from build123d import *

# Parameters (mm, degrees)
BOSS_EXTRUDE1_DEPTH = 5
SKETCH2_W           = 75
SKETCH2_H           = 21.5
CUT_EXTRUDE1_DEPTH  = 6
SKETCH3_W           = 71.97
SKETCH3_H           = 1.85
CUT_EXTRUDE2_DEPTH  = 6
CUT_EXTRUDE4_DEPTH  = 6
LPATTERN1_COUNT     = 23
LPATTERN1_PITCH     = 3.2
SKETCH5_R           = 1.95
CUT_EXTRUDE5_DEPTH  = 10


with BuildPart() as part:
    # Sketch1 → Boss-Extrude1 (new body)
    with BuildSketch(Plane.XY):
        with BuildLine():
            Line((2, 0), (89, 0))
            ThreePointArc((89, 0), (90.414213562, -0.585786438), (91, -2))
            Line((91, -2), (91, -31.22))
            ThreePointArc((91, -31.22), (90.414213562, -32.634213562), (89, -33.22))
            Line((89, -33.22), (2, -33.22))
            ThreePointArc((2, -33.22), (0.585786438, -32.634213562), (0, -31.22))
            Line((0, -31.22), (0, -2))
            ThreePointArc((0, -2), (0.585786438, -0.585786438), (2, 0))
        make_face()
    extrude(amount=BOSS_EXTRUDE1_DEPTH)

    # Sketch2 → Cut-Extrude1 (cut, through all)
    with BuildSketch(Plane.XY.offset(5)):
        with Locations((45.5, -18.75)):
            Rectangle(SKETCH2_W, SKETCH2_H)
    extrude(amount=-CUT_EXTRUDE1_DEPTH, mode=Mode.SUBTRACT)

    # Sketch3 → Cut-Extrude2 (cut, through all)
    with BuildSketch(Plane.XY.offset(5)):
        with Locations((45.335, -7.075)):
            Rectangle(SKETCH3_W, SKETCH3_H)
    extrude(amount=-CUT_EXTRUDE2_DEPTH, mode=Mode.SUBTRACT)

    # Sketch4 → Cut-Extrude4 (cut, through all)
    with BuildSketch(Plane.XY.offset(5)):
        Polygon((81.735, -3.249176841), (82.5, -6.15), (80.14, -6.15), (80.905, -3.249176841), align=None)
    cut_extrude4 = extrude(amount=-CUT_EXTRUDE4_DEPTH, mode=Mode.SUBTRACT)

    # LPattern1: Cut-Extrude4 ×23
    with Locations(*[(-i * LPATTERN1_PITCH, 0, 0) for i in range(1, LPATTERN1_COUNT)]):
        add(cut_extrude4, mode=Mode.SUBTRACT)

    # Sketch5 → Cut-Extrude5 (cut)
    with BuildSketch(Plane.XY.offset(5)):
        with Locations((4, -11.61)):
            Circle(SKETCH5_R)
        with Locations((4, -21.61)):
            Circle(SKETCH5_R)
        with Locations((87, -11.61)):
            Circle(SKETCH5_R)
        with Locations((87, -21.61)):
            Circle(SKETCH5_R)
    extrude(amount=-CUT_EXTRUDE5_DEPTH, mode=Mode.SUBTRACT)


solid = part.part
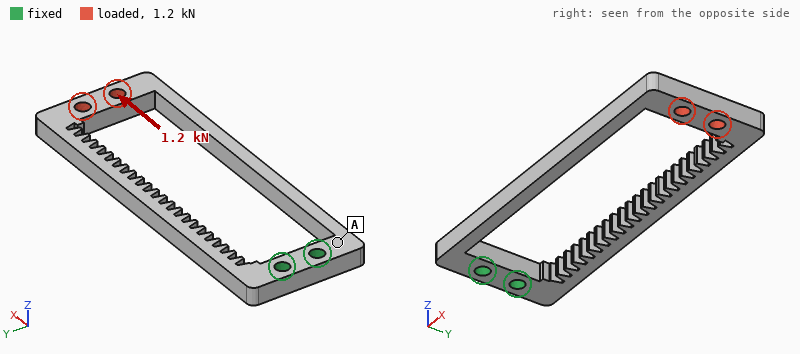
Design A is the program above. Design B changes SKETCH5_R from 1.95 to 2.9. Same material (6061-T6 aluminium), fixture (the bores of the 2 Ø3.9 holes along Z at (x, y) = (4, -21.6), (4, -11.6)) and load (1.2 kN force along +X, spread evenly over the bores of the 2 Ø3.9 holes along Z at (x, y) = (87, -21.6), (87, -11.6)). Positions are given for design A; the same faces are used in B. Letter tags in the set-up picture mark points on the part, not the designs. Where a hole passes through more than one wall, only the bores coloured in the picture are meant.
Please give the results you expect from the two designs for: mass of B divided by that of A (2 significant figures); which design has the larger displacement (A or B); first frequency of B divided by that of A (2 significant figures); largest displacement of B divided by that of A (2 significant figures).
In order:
0.95
B
1.1
1.2
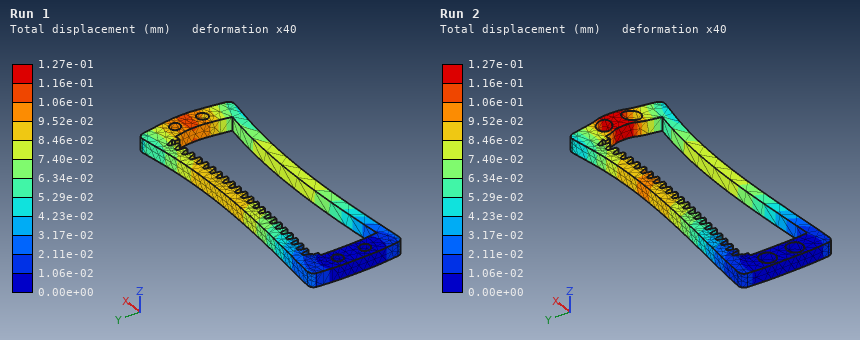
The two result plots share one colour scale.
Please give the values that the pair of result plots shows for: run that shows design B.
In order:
Run 2
